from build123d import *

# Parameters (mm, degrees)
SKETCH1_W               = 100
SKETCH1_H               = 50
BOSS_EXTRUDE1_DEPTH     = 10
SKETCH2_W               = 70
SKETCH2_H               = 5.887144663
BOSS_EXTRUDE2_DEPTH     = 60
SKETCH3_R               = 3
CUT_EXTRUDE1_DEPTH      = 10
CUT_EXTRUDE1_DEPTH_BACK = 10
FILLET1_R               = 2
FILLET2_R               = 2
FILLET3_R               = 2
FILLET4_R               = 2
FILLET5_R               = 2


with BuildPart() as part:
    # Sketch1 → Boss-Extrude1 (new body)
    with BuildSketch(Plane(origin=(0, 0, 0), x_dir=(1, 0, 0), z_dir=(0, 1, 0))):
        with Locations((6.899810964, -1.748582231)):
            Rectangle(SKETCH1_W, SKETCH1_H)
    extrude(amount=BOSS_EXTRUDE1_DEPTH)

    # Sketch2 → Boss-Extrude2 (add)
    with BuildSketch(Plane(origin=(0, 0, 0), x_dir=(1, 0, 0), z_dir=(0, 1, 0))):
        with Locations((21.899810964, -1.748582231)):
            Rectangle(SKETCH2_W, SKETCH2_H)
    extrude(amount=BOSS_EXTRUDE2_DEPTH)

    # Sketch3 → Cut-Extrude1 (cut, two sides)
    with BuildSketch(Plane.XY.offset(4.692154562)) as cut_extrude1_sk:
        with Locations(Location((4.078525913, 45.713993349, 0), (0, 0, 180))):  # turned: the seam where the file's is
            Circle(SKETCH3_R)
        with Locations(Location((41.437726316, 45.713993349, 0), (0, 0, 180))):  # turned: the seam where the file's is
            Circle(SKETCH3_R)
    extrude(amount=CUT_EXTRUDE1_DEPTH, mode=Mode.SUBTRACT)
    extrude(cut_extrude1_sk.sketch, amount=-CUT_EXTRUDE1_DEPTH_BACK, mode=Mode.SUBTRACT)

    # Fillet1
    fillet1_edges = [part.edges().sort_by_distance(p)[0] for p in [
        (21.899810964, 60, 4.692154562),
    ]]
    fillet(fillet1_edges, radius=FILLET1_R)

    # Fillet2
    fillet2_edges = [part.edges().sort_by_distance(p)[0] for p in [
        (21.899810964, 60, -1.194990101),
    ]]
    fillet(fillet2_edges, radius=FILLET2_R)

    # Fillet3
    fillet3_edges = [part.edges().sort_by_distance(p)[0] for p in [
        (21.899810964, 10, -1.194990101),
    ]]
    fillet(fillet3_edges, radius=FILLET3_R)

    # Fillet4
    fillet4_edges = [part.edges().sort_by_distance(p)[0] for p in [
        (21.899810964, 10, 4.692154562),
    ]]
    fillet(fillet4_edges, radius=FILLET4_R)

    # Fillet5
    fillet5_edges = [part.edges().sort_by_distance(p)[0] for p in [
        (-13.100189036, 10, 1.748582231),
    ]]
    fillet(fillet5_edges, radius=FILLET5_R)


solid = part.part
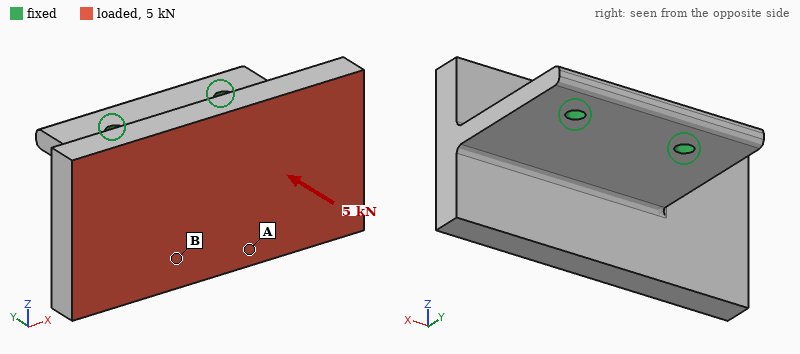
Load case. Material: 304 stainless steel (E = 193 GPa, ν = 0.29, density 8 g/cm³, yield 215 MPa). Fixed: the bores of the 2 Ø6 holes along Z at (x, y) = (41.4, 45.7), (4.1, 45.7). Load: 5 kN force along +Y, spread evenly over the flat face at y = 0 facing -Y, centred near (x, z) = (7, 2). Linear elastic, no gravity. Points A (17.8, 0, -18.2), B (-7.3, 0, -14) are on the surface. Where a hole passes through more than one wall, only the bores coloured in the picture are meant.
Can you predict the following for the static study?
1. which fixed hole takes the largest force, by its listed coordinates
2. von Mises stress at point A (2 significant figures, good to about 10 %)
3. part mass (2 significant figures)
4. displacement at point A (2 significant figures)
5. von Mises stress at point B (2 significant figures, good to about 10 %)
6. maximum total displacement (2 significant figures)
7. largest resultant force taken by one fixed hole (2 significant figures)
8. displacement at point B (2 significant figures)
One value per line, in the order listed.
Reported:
(4.1, 45.7)
7.7 MPa
560 g
5.8 µm
21 MPa
35 µm
4.5 kN
11 µm
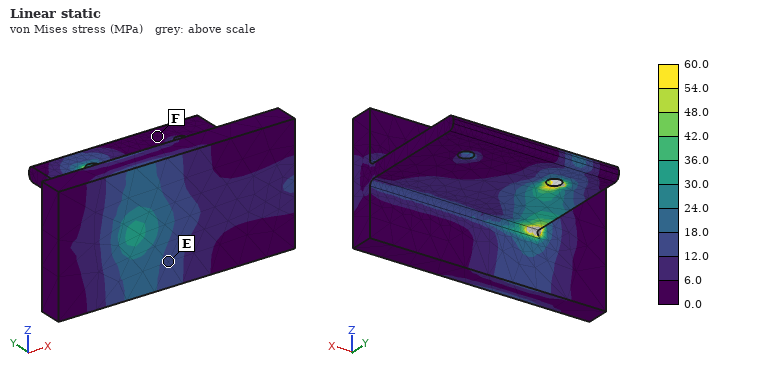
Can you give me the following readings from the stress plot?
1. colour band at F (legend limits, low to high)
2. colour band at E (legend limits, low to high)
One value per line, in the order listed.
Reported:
0.0 to 6.0 MPa
12.0 to 18.0 MPa
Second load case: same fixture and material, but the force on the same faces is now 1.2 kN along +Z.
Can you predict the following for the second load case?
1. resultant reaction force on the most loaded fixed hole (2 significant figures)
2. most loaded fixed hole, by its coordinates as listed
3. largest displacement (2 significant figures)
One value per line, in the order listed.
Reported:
1.0 kN
(4.1, 45.7)
0.26 mm
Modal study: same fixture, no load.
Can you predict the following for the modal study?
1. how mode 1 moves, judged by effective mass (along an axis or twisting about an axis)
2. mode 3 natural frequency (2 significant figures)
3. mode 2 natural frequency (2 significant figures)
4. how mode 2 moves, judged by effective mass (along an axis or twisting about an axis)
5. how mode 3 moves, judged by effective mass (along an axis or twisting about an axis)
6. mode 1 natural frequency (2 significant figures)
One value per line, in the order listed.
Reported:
along Z
3200 Hz
1200 Hz
twisting about Y
along Z
660 Hz
